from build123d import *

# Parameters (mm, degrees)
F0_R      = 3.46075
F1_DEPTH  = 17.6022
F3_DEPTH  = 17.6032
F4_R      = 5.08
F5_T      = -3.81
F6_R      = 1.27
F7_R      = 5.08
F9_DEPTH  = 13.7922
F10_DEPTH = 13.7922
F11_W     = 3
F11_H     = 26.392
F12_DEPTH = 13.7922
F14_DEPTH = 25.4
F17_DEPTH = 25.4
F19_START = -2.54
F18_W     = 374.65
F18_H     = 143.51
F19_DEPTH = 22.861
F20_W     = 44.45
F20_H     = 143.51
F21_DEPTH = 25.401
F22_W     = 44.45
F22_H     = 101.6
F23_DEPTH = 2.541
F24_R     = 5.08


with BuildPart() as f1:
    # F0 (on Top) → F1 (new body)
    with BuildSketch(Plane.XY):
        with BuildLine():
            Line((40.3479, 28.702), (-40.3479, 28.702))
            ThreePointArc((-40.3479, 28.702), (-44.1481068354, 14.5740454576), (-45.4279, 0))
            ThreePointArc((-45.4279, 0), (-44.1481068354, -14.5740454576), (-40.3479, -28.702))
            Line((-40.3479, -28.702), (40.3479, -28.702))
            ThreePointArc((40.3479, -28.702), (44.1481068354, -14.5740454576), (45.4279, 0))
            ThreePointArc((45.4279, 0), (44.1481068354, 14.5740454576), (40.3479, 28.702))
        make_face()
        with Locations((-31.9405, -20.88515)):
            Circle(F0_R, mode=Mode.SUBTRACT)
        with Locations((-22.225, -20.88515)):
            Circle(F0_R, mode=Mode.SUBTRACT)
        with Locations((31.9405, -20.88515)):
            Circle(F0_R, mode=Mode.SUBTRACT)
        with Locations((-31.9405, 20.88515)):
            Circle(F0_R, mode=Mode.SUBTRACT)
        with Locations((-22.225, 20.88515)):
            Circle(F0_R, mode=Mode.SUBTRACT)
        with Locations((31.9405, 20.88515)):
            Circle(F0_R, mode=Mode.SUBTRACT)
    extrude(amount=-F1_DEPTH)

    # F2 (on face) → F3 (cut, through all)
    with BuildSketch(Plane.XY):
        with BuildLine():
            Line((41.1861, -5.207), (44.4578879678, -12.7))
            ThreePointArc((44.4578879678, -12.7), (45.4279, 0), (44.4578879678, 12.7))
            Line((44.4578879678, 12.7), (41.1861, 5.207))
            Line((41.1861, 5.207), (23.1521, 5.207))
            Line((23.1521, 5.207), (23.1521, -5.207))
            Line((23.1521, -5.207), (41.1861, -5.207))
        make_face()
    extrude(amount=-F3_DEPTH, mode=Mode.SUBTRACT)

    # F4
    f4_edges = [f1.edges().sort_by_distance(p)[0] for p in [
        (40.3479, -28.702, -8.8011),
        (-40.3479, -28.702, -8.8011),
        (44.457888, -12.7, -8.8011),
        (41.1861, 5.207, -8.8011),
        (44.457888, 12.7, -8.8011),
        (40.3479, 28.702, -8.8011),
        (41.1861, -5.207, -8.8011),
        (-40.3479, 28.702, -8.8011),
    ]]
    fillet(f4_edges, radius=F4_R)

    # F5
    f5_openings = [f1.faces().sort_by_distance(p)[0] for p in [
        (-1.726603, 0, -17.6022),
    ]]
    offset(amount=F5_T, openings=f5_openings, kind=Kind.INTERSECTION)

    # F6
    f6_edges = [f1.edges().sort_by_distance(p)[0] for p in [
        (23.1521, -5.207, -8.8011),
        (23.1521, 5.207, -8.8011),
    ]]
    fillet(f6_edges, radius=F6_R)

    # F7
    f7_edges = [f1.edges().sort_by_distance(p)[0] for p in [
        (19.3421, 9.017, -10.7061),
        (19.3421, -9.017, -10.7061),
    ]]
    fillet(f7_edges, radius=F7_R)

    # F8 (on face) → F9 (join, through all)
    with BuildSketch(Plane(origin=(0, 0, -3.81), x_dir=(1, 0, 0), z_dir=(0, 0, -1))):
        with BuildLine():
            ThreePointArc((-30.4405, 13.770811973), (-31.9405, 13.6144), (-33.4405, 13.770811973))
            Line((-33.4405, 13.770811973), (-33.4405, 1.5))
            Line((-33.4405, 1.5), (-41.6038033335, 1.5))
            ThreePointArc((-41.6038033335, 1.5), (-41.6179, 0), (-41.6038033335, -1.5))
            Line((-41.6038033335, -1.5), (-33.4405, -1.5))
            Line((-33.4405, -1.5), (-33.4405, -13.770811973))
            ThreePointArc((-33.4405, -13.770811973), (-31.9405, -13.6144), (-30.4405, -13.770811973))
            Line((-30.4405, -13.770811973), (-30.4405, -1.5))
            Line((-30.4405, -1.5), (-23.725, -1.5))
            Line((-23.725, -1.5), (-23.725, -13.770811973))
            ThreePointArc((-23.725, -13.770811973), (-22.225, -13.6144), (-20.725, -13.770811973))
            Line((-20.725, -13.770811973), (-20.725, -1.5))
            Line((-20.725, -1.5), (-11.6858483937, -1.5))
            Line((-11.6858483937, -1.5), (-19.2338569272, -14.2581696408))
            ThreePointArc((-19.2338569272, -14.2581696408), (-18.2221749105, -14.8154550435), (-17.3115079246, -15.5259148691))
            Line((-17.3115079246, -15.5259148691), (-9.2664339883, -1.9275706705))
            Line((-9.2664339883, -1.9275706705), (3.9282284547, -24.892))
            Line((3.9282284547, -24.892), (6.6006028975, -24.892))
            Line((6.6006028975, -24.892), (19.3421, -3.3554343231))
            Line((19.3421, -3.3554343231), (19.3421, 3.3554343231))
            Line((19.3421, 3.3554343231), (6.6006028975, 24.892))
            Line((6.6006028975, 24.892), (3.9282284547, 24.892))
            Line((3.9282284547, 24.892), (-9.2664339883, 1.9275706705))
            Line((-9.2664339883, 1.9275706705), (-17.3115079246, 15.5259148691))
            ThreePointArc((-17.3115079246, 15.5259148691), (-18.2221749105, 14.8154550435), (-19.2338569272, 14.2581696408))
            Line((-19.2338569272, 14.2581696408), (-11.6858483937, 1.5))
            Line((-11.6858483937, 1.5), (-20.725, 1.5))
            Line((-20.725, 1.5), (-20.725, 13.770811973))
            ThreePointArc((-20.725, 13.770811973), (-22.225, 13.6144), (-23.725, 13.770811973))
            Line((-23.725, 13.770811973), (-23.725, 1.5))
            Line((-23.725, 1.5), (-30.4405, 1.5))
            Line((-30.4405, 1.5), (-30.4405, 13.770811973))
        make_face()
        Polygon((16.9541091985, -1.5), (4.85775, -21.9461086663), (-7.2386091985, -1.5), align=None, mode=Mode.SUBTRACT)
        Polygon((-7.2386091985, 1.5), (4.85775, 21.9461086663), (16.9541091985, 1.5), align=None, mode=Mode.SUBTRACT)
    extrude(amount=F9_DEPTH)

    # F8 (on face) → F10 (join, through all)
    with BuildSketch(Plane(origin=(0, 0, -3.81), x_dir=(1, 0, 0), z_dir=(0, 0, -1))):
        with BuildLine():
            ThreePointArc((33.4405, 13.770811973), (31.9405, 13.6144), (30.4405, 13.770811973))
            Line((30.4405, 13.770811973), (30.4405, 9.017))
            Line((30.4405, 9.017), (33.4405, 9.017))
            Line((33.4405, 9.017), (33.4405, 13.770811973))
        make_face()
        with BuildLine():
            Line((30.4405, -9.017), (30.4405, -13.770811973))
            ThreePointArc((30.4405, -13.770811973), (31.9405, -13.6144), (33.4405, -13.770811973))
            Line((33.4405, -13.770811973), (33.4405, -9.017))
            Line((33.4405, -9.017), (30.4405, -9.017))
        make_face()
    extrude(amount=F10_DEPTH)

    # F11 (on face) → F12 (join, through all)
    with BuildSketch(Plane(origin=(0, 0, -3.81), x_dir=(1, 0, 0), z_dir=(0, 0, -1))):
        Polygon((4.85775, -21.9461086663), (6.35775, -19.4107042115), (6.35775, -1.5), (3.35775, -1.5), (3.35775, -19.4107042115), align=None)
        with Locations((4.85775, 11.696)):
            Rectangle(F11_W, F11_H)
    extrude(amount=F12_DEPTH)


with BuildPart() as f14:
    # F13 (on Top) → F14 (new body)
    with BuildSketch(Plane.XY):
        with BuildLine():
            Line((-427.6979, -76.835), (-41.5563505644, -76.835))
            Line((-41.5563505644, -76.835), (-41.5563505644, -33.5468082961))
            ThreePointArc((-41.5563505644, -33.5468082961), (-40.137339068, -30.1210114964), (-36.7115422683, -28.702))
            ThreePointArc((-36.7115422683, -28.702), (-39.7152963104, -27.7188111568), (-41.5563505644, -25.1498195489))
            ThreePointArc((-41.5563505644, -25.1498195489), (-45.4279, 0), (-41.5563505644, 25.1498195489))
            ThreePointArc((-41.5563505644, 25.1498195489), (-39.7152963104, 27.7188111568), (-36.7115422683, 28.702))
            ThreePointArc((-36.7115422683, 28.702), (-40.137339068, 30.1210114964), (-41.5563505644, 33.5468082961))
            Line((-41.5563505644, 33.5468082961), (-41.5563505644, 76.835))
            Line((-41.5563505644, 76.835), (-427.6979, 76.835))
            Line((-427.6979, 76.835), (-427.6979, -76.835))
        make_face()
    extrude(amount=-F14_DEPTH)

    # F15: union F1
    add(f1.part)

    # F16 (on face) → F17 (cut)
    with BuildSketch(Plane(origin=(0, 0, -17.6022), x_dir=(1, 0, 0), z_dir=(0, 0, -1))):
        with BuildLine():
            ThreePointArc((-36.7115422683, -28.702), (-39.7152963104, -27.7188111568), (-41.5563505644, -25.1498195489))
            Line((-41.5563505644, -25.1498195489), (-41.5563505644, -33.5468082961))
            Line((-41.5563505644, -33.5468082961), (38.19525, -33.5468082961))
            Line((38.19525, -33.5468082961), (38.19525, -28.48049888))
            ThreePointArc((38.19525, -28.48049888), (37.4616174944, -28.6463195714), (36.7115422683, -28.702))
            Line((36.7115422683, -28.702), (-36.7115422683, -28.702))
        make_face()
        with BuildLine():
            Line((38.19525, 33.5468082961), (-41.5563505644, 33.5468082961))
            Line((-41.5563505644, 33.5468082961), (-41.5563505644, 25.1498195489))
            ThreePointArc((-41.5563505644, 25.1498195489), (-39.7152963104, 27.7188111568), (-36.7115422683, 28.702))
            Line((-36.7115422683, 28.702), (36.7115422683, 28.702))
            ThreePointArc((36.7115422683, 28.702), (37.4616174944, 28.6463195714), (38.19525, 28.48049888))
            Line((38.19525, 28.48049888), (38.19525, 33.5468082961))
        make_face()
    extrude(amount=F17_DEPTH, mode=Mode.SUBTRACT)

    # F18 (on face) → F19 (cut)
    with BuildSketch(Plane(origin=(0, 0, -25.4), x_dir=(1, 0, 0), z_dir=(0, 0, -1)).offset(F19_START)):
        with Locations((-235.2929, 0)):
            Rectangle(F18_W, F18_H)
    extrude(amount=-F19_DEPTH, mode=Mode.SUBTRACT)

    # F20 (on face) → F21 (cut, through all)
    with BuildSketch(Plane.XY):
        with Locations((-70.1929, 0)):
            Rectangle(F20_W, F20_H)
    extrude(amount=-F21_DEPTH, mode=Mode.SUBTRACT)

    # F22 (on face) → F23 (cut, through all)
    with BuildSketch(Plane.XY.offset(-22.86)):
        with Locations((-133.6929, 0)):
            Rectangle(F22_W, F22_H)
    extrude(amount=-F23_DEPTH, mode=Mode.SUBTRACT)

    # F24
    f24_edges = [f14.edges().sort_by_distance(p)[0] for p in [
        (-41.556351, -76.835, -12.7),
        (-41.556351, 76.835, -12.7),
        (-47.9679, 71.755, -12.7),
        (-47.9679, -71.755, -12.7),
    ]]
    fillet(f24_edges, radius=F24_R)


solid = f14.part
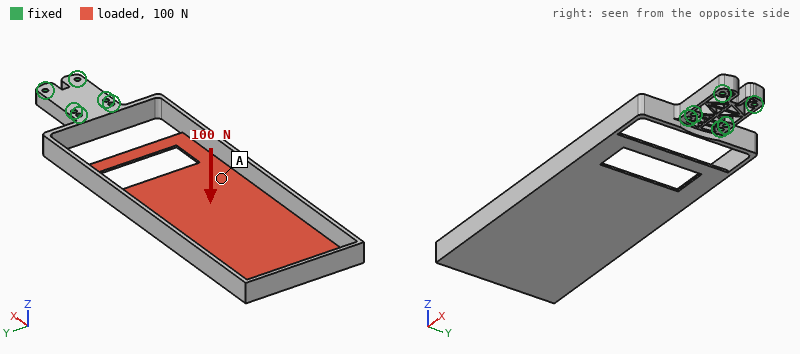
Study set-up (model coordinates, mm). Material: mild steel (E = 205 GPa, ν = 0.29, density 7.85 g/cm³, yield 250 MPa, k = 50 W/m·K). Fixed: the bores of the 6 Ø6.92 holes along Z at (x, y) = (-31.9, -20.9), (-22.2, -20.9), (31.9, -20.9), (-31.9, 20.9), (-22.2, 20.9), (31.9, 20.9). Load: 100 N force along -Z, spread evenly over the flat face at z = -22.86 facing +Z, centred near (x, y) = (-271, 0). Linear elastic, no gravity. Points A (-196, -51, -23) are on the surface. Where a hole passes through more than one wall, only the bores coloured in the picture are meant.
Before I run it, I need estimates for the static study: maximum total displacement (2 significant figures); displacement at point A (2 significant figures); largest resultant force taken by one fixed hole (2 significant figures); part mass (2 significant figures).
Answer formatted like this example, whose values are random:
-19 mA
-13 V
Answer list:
1.4 mm
0.54 mm
120 N
2.3 kg
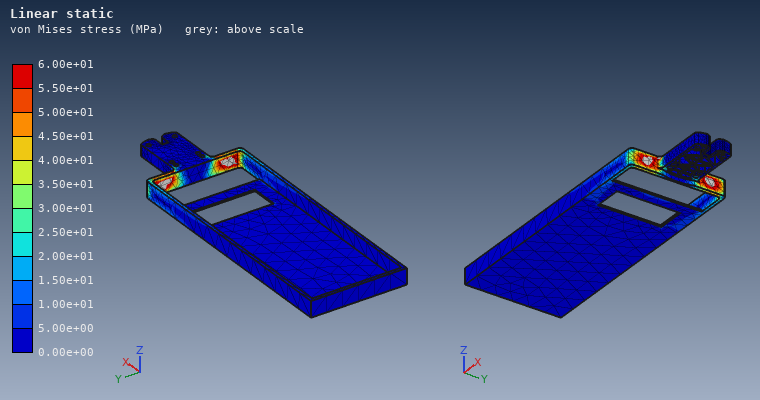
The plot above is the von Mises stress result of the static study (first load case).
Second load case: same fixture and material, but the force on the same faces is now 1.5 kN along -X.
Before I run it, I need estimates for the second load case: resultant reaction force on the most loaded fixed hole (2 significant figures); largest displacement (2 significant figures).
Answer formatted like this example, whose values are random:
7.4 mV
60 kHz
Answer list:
1.6 kN
1.0 mm
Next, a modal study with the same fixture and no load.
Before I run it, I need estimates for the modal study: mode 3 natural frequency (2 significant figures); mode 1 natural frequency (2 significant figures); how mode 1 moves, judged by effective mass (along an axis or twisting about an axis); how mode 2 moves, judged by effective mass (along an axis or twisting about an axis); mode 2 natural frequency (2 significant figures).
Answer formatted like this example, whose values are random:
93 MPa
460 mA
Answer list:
110 Hz
38 Hz
along Z
along Y
72 Hz
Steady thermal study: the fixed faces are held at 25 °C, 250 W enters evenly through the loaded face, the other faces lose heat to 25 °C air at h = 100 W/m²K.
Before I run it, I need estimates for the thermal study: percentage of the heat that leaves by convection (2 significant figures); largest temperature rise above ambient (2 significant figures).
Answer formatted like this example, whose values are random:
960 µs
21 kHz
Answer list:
100 %
49 K
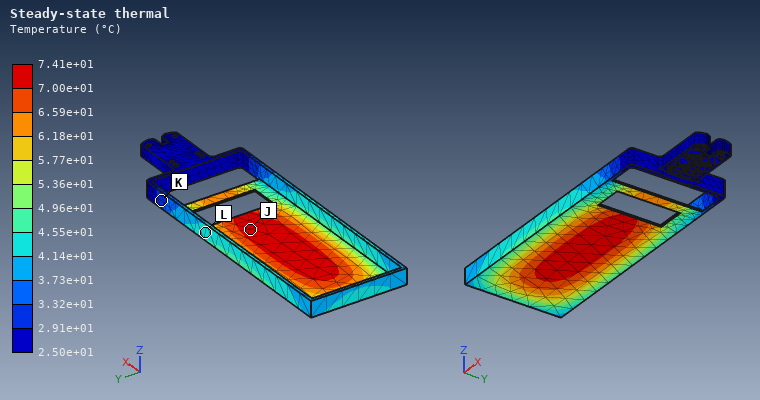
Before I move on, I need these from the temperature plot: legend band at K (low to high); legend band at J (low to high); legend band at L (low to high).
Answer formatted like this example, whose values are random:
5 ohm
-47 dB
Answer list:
2.91e+01 to 3.32e+01 °C
7.00e+01 to 7.41e+01 °C
4.14e+01 to 4.55e+01 °C
